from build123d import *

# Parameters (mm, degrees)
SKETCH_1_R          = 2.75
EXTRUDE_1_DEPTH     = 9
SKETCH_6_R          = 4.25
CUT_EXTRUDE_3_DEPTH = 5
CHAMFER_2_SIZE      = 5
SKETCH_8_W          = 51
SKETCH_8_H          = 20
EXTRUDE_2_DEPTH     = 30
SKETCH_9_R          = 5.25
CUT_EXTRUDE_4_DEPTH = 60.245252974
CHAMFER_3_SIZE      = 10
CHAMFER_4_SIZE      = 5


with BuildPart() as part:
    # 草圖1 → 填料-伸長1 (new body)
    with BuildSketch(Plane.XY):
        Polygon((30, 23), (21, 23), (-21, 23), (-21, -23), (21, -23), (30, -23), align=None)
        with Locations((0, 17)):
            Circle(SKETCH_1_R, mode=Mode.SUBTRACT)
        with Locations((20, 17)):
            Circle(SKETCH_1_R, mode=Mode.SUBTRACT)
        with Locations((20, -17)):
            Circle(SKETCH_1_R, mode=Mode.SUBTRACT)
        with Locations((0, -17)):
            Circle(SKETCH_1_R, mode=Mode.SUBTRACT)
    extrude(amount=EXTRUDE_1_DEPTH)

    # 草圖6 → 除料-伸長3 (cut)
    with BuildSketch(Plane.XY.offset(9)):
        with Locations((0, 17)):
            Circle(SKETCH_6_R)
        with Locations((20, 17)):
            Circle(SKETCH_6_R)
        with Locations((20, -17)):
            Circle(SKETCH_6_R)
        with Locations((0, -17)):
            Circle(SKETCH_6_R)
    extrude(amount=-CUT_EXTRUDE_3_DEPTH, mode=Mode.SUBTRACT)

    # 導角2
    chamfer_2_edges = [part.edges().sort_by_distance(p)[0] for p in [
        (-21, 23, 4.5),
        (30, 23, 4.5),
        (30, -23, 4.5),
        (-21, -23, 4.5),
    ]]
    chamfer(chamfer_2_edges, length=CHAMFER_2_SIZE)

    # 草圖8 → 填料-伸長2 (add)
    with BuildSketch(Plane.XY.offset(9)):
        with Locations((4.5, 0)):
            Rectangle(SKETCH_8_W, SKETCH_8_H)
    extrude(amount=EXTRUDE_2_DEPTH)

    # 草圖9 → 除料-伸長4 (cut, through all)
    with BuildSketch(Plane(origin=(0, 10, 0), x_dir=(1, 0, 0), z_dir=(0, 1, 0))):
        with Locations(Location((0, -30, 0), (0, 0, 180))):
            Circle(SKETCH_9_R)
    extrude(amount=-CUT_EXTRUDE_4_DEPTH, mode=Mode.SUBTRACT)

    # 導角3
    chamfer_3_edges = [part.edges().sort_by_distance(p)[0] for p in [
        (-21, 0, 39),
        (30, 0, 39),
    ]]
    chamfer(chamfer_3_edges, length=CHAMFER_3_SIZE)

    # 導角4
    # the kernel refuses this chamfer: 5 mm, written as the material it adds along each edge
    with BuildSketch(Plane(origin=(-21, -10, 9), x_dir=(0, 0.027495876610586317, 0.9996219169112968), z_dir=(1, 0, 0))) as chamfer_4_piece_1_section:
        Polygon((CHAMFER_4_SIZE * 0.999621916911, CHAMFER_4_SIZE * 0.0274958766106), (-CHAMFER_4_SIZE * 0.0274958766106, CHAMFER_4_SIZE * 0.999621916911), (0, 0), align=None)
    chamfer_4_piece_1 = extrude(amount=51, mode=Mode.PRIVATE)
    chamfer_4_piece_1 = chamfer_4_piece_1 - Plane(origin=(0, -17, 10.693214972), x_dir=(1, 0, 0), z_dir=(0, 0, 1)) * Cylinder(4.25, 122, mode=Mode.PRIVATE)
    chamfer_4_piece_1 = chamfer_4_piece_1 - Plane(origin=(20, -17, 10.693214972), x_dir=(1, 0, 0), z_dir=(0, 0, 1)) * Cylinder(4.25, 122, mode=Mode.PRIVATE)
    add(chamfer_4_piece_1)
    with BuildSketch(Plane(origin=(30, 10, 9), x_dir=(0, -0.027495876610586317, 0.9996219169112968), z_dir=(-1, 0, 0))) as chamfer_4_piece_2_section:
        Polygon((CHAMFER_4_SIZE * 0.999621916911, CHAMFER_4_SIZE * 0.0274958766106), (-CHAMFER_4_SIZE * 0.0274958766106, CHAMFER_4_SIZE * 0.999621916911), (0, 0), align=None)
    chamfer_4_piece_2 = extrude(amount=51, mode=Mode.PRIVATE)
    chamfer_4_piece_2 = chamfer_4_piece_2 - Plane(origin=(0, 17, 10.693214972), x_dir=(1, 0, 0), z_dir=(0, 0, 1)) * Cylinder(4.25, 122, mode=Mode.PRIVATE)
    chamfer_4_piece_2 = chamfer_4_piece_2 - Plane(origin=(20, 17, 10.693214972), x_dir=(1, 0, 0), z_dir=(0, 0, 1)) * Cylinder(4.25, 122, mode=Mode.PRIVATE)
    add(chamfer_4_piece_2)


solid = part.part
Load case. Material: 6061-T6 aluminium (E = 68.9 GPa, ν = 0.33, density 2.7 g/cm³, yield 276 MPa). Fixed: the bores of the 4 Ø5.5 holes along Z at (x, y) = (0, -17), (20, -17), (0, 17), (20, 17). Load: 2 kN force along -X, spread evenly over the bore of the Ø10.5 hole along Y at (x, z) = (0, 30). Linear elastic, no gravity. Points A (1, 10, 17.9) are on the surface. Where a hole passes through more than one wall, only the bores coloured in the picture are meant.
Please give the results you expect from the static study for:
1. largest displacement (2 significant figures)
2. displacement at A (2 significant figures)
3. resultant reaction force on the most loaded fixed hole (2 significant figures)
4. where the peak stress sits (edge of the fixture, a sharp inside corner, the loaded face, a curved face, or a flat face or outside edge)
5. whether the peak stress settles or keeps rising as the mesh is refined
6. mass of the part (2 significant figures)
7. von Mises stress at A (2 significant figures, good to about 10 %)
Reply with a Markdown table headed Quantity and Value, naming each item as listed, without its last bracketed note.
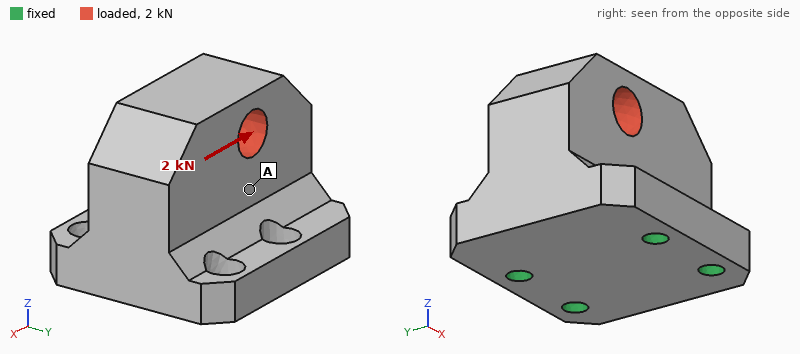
| Quantity | Value |
|---|---|
| largest displacement | 24 µm |
| displacement at A | 10 µm |
| resultant reaction force on the most loaded fixed hole | 1.4 kN |
| where the peak stress sits | edge of the fixture |
| whether the peak stress settles or keeps rising as the mesh is refined | keeps rising |
| mass of the part | 130 g |
| von Mises stress at A | 8.1 MPa |
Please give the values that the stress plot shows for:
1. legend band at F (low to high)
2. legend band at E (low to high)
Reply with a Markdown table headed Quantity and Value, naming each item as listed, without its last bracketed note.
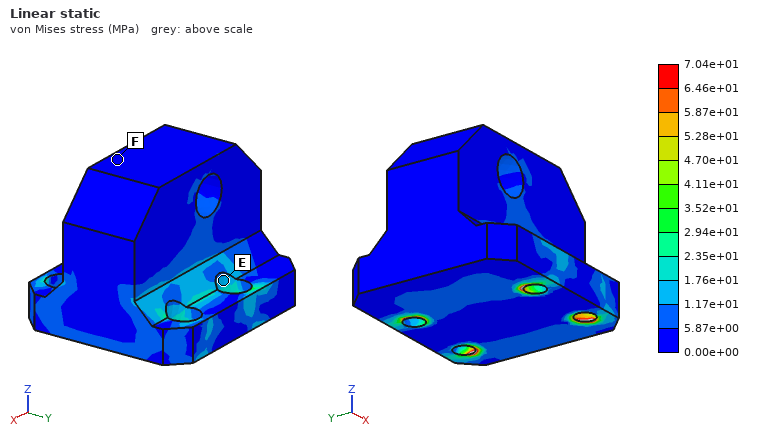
| Quantity | Value |
|---|---|
| legend band at F | 0.00e+00 to 5.87e+00 MPa |
| legend band at E | 1.17e+01 to 1.76e+01 MPa |
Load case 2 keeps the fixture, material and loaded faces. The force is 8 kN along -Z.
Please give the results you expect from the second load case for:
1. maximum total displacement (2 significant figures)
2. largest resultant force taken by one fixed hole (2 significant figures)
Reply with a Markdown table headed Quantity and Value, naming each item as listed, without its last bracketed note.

| Quantity | Value |
|---|---|
| maximum total displacement | 35 µm |
| largest resultant force taken by one fixed hole | 4.0 kN |
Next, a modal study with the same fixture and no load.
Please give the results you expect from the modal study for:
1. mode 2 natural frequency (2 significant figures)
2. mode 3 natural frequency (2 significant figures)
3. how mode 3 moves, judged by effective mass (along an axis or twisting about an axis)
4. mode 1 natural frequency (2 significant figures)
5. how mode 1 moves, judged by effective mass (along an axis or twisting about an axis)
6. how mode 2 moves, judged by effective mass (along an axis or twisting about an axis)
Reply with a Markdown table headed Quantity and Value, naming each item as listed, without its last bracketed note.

| Quantity | Value |
|---|---|
| mode 2 natural frequency | 10 kHz |
| mode 3 natural frequency | 15 kHz |
| how mode 3 moves, judged by effective mass | along Z |
| mode 1 natural frequency | 6400 Hz |
| how mode 1 moves, judged by effective mass | along X |
| how mode 2 moves, judged by effective mass | along Y |
